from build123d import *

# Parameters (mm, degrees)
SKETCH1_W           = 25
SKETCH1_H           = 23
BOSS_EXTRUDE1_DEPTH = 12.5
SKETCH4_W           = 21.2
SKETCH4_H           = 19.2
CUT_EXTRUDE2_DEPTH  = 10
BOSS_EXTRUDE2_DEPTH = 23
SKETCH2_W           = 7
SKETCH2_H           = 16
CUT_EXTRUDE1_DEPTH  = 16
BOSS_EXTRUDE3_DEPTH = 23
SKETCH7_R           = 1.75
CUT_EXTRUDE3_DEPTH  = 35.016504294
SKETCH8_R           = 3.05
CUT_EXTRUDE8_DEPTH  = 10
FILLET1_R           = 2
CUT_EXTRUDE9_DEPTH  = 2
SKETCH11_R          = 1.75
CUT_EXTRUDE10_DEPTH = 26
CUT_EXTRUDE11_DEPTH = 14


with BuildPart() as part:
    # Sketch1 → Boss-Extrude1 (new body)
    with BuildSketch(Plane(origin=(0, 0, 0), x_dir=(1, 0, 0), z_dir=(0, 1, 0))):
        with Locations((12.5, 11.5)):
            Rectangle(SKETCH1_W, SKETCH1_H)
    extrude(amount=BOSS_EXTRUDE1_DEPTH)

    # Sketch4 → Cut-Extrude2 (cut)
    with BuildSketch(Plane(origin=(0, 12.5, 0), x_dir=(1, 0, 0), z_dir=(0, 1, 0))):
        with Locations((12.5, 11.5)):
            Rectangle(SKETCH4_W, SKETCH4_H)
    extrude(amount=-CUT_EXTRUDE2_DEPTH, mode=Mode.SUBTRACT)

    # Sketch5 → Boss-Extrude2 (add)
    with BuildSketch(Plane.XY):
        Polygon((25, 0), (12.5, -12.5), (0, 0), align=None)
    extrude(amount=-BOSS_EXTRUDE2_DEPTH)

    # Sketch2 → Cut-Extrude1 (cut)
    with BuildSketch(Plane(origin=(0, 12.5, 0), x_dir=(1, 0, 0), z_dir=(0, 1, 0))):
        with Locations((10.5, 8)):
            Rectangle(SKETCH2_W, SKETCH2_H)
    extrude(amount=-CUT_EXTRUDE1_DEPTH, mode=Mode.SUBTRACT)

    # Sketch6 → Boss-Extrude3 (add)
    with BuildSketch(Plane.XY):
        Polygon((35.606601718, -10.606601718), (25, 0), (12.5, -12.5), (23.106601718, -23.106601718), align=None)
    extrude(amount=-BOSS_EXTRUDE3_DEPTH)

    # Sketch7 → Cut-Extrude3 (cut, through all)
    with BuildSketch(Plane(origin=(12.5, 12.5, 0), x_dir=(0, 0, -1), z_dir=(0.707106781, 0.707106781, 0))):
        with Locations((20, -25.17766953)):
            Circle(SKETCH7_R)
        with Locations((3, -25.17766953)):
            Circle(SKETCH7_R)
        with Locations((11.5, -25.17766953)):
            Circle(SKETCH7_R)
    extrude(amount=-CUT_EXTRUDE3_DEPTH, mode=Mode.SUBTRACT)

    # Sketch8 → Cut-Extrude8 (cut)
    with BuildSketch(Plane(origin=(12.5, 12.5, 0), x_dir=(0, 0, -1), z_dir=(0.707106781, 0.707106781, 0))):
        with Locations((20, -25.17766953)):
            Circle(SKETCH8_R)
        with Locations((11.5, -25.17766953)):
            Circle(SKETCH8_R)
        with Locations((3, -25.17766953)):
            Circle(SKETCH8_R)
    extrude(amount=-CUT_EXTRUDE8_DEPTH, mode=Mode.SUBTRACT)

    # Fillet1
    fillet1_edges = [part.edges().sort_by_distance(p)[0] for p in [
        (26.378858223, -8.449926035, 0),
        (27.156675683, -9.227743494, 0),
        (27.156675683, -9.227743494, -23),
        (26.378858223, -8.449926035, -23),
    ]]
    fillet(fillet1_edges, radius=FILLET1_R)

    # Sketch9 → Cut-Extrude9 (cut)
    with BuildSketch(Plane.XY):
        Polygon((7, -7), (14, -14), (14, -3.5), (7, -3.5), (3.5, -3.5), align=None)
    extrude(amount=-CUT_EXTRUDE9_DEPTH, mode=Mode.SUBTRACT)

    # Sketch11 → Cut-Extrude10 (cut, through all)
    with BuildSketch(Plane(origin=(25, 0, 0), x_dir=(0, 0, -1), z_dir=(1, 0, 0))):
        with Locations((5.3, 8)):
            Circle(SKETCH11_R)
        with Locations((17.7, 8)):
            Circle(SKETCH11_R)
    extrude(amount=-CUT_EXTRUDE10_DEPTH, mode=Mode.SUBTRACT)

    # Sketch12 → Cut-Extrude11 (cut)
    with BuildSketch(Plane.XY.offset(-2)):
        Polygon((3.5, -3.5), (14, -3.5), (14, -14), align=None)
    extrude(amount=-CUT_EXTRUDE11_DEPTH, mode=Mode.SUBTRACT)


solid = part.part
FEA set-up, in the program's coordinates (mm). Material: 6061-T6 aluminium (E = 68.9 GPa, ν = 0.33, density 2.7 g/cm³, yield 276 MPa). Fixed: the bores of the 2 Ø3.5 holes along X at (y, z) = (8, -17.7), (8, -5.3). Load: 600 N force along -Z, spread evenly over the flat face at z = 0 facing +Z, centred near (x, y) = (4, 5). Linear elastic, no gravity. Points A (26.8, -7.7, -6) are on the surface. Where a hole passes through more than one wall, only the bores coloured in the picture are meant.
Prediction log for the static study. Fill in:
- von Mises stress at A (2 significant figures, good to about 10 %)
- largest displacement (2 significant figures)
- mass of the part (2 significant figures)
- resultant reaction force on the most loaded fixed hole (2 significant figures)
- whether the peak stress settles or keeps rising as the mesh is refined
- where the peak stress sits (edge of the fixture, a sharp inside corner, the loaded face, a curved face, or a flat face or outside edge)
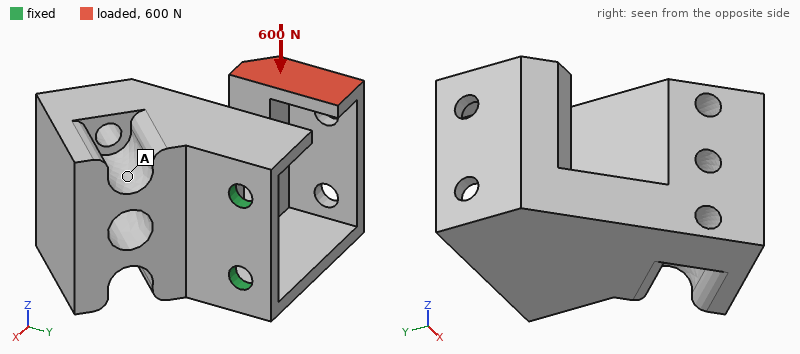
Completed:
27 MPa
0.20 mm
27 g
780 N
keeps rising
edge of the fixture
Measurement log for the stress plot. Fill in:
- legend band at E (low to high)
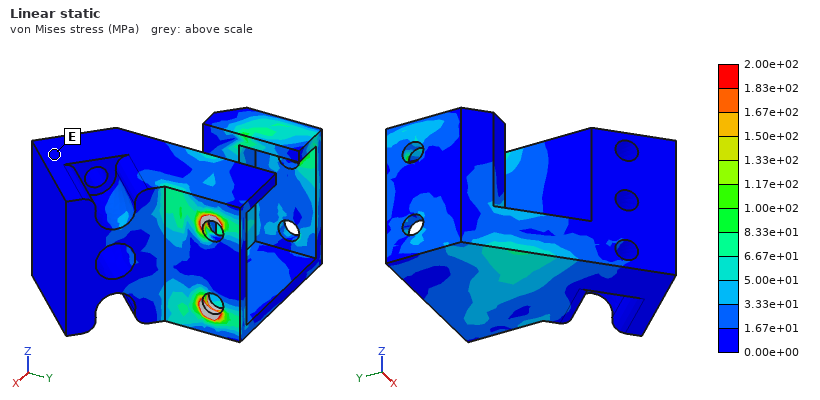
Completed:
0.00e+00 to 1.67e+01 MPa
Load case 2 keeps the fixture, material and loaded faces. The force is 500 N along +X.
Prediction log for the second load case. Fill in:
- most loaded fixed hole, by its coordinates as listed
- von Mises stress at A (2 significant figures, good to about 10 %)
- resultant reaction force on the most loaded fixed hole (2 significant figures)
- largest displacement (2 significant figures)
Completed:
(8, -5.3)
21 MPa
580 N
0.40 mm
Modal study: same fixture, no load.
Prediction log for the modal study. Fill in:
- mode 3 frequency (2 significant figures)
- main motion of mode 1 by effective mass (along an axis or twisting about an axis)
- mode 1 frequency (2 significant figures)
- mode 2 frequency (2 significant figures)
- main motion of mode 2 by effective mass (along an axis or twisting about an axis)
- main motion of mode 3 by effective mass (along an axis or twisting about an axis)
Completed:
6300 Hz
along X
1500 Hz
4500 Hz
along Z
along X
